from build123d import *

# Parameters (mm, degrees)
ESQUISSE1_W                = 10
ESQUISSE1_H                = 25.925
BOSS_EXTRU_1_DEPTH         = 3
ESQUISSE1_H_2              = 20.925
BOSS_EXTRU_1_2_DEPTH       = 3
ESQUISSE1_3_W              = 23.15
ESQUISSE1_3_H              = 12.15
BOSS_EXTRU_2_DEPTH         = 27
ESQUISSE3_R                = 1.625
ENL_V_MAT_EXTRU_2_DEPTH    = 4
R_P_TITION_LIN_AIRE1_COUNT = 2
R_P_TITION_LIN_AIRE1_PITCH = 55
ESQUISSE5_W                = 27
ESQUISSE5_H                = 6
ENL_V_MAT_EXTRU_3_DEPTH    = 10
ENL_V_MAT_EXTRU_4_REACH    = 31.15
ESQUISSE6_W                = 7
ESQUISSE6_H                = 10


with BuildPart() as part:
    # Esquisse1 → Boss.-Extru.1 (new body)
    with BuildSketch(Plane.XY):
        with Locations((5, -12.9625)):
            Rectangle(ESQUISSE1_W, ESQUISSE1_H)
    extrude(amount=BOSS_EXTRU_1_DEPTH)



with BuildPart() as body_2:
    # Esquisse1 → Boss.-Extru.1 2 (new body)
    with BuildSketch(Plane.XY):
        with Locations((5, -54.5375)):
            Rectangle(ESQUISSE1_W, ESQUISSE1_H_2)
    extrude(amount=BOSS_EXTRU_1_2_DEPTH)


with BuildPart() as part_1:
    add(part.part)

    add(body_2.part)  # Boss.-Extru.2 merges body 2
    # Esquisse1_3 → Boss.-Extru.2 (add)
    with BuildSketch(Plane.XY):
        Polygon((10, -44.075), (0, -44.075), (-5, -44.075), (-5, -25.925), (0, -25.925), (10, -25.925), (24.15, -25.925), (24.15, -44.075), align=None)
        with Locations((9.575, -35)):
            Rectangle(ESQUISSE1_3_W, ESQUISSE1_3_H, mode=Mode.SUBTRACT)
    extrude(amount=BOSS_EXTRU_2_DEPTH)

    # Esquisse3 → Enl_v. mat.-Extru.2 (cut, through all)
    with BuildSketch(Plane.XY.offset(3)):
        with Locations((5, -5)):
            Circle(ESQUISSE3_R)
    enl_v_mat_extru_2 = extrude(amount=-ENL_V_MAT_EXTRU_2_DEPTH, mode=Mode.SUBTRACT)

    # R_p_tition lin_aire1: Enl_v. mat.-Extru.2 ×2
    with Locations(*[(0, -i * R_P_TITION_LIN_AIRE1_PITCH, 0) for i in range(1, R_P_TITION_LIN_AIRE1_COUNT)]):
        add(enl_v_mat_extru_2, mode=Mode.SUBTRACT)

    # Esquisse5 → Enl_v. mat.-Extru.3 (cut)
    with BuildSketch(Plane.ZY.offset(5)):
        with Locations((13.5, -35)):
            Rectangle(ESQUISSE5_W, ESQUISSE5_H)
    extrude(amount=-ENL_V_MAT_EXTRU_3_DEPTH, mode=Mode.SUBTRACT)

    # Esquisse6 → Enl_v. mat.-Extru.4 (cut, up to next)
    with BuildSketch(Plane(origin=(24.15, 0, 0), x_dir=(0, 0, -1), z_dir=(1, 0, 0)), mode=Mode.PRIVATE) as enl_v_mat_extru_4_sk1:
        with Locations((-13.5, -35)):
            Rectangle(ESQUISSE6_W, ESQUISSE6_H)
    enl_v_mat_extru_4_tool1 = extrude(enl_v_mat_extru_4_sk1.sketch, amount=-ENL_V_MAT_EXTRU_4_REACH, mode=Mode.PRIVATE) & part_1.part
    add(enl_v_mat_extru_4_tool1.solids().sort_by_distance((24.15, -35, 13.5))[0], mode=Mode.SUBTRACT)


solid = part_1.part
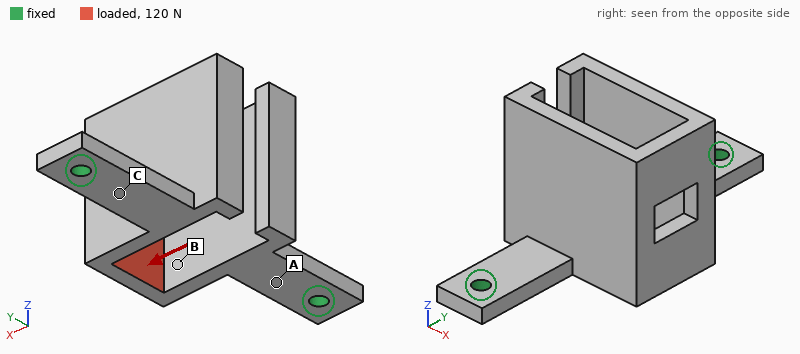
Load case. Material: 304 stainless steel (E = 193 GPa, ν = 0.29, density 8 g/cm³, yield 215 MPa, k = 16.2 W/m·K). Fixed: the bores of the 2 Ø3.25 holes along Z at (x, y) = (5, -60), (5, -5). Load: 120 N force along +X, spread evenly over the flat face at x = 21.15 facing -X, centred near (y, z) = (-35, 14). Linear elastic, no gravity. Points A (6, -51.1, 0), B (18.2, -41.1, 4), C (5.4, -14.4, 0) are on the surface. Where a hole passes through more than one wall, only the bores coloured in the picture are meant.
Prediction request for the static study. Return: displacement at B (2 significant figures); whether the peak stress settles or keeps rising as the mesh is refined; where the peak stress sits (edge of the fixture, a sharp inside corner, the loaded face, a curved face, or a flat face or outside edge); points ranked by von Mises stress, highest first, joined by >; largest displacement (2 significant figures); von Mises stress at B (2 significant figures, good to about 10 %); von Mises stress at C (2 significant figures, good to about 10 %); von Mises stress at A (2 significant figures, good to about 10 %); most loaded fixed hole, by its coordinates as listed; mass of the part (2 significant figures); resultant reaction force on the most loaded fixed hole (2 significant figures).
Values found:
31 µm
keeps rising
edge of the fixture
A > C > B
75 µm
6.4 MPa
37 MPa
49 MPa
(5, -60)
59 g
70 N
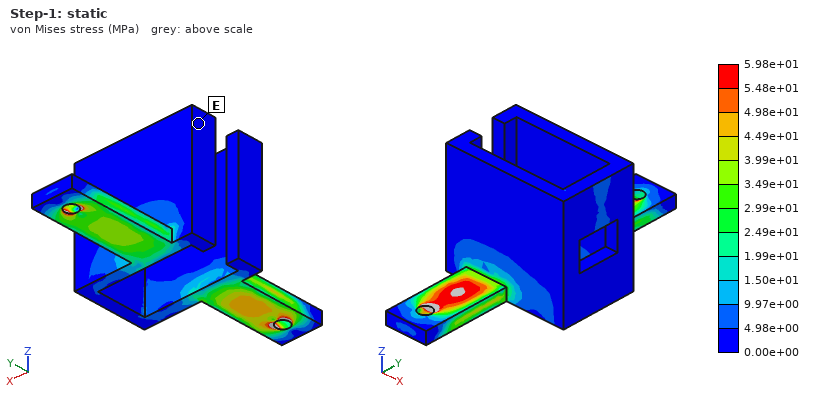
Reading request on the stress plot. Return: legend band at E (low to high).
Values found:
0.00e+00 to 4.98e+00 MPa
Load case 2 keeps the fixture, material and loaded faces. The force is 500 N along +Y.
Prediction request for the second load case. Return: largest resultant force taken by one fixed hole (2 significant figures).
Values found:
360 N
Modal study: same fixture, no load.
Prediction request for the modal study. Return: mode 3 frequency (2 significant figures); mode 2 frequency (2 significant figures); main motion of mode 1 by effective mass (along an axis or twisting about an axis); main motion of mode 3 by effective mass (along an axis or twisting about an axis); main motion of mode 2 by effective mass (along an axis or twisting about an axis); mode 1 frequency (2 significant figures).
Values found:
2400 Hz
2100 Hz
along X
along Y
along Z
1000 Hz
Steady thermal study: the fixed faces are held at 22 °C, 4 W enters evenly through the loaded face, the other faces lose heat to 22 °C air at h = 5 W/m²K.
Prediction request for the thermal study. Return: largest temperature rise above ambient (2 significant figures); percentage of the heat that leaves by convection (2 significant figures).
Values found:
87 K
38 %
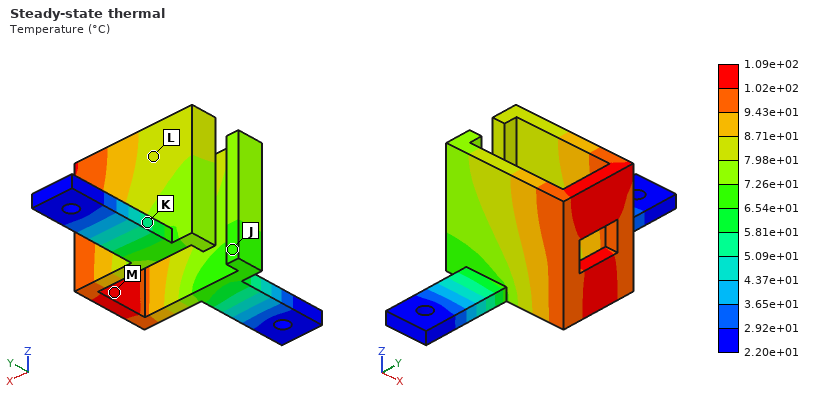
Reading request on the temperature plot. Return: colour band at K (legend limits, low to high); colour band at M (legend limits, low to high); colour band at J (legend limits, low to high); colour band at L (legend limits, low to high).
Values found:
5.09e+01 to 5.81e+01 °C
1.02e+02 to 1.09e+02 °C
6.54e+01 to 7.26e+01 °C
7.98e+01 to 8.71e+01 °C
